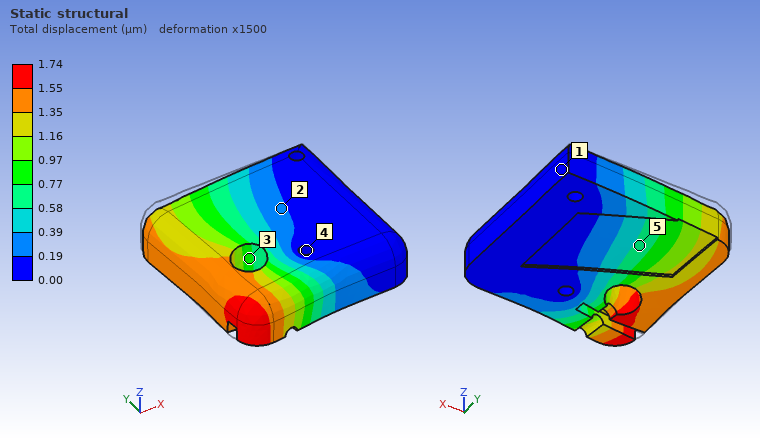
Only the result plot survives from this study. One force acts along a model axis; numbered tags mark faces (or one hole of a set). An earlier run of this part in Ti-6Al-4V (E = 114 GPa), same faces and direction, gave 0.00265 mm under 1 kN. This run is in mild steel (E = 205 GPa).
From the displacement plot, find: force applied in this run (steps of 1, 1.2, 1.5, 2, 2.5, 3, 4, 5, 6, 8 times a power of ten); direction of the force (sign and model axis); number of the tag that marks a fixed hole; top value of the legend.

1.2 kN
-Y
4
1.74 µm
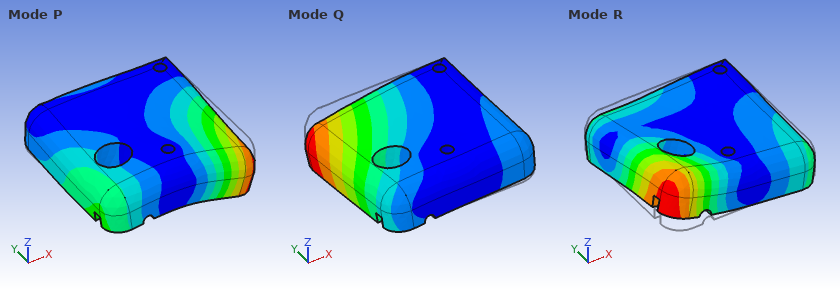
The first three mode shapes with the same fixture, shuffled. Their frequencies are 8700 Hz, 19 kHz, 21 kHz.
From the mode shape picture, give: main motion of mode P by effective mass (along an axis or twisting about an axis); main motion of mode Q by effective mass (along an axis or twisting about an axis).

along Z
along Z
